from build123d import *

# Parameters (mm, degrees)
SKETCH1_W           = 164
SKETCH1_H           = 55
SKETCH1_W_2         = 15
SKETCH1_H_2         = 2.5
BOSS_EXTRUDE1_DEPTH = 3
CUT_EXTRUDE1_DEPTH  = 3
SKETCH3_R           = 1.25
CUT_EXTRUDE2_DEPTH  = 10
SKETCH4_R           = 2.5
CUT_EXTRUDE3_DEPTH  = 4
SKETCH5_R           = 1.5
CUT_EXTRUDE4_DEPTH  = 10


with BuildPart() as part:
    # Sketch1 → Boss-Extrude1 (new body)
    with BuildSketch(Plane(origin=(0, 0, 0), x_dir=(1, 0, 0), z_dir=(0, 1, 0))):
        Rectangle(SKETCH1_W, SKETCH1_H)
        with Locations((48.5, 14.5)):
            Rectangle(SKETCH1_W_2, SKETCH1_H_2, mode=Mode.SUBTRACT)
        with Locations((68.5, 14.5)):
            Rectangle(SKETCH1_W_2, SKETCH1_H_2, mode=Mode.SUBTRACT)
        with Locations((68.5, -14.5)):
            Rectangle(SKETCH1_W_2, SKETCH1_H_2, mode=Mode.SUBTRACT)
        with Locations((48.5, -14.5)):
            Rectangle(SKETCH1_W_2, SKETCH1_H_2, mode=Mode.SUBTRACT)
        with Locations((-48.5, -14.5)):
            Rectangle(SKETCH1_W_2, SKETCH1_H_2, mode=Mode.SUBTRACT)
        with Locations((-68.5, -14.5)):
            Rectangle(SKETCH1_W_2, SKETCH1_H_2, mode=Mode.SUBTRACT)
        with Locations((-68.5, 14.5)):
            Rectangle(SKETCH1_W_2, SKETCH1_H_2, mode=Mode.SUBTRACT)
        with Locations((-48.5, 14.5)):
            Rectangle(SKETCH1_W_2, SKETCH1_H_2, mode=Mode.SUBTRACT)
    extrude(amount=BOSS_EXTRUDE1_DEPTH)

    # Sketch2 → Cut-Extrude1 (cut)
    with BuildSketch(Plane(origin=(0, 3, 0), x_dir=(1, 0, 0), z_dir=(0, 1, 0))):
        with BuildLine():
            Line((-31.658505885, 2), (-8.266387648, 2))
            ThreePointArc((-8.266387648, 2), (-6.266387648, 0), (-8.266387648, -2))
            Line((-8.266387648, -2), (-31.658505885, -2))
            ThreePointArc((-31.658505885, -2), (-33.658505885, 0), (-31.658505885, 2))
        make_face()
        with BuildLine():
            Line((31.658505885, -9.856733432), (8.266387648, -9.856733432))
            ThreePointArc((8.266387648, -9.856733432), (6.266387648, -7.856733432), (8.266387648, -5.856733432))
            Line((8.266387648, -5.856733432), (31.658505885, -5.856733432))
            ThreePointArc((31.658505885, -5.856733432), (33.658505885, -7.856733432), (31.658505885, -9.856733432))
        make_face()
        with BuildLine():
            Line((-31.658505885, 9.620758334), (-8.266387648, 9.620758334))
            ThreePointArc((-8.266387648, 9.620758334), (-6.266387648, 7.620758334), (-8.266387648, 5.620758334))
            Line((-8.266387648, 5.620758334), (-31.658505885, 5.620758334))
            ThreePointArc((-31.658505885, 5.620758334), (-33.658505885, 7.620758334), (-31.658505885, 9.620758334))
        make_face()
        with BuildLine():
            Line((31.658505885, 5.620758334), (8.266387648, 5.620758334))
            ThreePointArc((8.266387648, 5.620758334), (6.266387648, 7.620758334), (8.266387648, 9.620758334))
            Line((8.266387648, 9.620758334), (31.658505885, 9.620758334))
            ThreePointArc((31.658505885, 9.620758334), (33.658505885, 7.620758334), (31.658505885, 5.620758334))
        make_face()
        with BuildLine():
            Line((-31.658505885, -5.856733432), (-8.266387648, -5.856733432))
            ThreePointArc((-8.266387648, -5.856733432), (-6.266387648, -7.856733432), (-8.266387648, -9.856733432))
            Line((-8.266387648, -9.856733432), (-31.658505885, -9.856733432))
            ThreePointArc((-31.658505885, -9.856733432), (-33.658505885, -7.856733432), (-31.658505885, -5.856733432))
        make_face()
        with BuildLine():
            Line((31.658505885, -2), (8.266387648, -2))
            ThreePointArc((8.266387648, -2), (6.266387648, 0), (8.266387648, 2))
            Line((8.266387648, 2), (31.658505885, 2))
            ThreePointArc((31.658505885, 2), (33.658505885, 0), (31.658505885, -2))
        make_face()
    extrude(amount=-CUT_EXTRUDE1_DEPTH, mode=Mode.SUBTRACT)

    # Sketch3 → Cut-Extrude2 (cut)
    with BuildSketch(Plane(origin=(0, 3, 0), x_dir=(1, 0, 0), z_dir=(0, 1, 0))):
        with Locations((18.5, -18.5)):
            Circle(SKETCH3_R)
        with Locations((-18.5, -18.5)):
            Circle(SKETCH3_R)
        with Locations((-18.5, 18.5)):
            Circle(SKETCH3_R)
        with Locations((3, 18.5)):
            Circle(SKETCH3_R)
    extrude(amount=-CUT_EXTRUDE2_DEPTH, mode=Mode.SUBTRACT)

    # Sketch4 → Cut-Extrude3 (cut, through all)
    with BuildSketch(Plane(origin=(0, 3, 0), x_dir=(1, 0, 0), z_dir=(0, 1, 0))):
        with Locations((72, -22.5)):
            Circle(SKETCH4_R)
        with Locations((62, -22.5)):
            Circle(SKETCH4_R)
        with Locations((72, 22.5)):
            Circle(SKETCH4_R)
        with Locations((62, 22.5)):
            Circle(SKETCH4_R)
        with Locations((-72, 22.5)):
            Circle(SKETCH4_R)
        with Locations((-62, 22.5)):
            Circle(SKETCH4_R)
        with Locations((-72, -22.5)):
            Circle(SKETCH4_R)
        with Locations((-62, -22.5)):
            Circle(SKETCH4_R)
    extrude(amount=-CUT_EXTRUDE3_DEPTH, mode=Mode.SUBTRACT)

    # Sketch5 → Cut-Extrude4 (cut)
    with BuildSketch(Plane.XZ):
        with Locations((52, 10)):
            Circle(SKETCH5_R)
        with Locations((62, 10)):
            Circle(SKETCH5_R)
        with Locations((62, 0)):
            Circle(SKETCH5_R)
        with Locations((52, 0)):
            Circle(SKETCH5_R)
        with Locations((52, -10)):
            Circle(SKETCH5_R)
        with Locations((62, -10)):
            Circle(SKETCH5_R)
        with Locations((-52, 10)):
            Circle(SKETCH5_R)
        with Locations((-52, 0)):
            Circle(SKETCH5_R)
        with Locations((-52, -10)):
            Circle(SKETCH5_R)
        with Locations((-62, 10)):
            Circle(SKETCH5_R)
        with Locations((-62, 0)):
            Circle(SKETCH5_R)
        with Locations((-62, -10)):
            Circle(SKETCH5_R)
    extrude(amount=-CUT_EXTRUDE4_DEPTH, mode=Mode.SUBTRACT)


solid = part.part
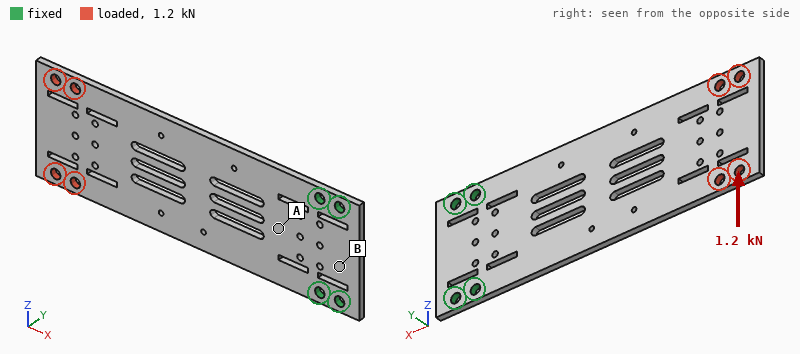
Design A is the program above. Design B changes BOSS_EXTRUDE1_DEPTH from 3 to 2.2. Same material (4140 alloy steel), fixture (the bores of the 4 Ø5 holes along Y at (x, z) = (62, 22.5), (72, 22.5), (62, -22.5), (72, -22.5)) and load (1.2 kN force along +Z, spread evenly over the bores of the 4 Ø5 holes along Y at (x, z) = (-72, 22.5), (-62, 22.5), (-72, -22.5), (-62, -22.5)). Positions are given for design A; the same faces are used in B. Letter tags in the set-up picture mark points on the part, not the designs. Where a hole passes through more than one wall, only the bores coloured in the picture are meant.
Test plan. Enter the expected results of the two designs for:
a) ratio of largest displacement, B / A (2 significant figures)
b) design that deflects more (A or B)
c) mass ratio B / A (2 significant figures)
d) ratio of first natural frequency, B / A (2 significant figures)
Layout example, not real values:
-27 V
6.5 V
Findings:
1.4
B
0.73
0.74
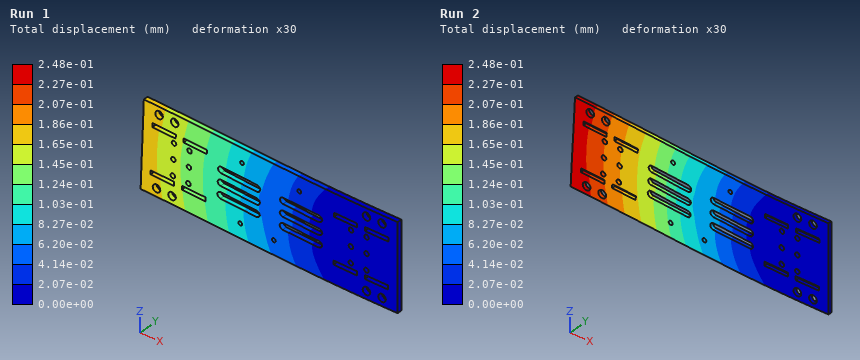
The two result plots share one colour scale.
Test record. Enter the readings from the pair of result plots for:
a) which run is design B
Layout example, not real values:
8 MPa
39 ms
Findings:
Run 2
